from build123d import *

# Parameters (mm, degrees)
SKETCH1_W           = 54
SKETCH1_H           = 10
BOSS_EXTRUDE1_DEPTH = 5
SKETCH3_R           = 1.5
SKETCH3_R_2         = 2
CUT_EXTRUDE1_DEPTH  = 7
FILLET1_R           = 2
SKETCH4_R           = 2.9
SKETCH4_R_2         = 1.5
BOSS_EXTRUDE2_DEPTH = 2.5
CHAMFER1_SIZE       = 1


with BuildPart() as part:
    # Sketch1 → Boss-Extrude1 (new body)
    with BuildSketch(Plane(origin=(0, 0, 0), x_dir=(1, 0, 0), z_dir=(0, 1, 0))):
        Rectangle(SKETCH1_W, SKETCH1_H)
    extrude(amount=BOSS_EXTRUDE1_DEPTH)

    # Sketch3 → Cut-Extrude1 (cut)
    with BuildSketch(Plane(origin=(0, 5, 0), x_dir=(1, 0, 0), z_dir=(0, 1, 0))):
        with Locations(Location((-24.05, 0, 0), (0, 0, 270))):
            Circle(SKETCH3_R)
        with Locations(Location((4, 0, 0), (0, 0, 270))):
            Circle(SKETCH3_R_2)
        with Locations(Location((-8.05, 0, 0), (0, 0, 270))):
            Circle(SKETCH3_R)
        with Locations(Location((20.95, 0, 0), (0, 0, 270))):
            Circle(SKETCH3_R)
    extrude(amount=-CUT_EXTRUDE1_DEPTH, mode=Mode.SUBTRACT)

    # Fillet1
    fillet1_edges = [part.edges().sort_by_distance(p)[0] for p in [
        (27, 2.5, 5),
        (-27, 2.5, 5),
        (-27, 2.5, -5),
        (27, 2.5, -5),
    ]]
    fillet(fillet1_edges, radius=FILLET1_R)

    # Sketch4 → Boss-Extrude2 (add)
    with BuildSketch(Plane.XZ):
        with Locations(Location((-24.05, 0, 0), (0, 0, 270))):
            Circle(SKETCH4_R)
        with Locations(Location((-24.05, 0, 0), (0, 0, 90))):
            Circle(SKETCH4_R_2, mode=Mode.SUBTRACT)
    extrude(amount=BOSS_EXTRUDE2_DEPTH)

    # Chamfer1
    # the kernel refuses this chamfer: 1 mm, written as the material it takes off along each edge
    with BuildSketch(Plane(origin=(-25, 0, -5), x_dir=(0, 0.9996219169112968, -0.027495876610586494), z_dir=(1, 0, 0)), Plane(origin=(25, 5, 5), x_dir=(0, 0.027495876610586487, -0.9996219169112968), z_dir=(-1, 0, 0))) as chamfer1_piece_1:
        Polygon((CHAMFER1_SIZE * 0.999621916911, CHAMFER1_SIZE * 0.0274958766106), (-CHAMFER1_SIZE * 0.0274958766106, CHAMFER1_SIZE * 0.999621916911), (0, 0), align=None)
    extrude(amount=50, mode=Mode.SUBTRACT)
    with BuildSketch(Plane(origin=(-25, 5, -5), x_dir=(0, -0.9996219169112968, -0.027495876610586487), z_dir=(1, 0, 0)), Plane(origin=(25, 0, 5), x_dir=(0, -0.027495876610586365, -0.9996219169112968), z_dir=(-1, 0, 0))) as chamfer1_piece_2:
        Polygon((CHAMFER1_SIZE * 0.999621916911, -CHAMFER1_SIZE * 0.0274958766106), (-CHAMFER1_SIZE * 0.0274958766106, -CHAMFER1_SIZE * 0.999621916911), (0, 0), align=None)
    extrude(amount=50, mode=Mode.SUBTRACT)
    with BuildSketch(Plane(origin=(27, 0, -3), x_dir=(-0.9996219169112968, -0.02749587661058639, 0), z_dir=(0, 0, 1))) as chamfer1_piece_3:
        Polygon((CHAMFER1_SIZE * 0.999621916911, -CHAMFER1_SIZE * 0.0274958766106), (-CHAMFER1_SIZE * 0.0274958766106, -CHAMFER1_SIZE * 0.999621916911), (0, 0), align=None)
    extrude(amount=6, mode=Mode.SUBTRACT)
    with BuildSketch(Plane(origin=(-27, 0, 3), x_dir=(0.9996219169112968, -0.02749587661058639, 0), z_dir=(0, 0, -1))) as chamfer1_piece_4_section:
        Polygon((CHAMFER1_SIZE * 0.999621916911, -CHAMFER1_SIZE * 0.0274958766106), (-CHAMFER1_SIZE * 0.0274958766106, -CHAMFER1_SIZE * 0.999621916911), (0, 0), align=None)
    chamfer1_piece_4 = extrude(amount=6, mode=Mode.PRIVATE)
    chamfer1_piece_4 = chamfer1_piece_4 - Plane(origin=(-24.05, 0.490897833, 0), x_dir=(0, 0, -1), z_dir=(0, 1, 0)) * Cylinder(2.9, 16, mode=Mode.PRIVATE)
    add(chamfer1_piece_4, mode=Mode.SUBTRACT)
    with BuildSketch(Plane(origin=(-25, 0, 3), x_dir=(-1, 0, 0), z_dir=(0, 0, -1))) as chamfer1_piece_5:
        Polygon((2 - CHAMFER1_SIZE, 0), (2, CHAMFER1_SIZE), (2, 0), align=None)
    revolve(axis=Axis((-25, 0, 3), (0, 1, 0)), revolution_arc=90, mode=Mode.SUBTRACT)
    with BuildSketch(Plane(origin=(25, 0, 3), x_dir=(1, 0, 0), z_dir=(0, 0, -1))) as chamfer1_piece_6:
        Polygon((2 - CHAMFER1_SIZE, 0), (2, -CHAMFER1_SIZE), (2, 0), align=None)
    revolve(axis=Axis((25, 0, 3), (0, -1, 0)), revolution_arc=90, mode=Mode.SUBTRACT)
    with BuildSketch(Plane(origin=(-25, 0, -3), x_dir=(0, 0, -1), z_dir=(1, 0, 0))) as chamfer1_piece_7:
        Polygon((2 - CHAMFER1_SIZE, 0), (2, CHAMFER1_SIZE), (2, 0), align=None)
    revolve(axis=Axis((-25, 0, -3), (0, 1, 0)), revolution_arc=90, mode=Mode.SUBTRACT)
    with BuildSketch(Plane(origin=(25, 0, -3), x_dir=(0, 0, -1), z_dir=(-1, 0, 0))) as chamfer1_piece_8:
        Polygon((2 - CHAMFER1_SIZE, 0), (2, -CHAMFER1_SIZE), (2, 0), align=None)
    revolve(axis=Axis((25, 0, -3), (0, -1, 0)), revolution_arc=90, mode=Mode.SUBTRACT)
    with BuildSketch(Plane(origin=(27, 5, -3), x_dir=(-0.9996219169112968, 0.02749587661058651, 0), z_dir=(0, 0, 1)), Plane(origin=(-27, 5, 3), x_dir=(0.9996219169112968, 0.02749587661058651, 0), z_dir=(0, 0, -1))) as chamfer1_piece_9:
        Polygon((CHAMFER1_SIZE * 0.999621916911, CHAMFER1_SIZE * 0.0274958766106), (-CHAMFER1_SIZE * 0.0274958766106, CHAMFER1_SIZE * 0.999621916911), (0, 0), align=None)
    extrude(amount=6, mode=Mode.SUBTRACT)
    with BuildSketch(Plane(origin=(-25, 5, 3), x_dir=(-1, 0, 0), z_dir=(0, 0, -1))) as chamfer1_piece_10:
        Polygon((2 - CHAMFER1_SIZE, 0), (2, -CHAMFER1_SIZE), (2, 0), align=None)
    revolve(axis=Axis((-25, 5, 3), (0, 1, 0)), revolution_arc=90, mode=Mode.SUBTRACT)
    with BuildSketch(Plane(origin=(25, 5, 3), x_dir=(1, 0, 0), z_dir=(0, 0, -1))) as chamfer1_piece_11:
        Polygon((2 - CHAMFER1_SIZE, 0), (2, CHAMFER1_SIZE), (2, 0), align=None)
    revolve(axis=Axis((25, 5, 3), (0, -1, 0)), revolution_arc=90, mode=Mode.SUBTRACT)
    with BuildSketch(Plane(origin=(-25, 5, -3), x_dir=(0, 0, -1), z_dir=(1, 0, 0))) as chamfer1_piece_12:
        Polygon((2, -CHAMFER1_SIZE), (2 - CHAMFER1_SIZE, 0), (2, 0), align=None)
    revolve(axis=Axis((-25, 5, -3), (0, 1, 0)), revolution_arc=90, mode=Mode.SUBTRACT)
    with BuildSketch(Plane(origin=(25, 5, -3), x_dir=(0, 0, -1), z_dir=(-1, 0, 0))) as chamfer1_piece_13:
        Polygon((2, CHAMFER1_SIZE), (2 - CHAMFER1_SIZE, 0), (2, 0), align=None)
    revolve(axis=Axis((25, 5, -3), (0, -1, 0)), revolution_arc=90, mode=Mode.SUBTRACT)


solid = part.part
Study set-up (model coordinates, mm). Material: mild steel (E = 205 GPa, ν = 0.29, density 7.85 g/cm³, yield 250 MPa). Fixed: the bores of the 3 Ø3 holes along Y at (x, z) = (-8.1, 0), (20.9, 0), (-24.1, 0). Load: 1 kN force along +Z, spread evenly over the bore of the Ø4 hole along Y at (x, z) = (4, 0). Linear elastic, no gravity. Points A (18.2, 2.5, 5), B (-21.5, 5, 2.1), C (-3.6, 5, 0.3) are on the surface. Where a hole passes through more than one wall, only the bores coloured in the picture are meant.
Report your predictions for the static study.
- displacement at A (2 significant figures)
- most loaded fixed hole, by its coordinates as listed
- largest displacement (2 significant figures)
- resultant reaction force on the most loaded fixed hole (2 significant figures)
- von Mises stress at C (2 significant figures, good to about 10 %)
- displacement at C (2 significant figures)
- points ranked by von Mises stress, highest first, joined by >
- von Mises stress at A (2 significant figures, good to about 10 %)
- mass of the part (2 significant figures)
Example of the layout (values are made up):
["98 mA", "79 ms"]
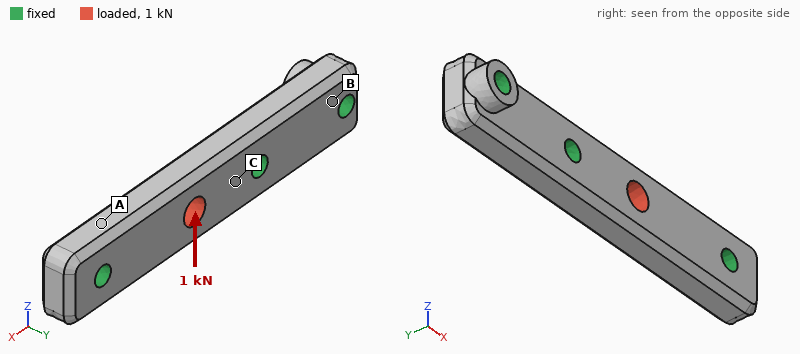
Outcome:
["1.3 µm", "(-8.1, 0)", "4.5 µm", "710 N", "33 MPa", "1.4 µm", "C > A > B", "18 MPa", "19 g"]
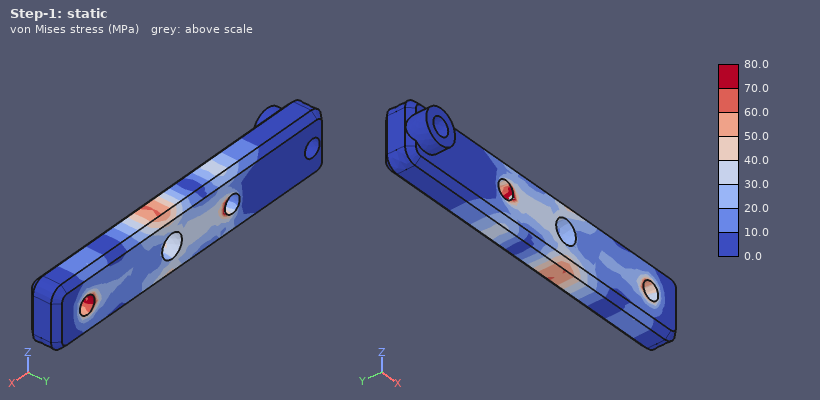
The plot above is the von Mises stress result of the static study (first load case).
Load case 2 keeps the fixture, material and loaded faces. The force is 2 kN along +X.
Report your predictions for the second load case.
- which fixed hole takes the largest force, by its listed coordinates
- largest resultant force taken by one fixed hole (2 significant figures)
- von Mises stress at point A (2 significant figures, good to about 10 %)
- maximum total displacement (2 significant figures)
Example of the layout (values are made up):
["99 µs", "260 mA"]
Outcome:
["(-8.1, 0)", "1.1 kN", "10.0 MPa", "1.6 µm"]
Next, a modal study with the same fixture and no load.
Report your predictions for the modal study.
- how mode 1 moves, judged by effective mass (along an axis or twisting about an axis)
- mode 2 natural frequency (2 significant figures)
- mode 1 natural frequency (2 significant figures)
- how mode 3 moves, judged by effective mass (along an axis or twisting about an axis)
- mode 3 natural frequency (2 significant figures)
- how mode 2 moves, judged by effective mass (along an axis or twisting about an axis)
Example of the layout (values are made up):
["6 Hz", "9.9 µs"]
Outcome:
["along Y", "35 kHz", "27 kHz", "twisting about X", "44 kHz", "along Z"]
